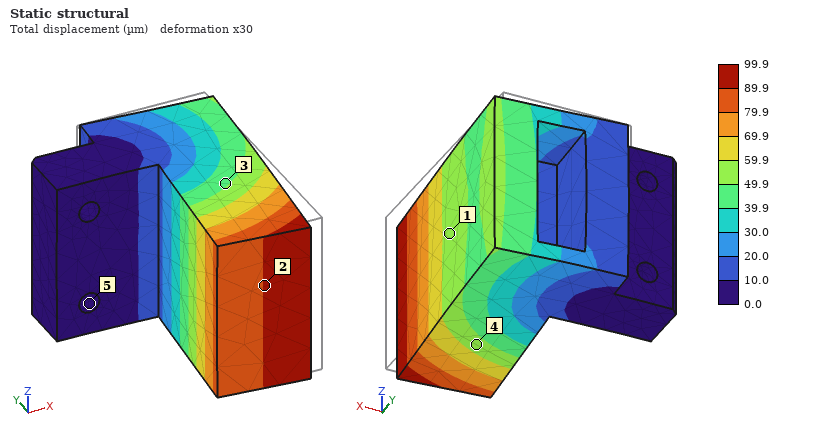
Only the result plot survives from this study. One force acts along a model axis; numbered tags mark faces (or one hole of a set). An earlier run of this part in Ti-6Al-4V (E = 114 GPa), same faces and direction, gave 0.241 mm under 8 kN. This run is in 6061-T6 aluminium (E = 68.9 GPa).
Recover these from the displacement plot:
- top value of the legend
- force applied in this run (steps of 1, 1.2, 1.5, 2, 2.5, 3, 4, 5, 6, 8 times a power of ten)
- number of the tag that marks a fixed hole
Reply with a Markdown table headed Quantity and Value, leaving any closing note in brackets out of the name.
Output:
| Quantity | Value |
|---|---|
| top value of the legend | 99.9 µm |
| force applied in this run | 2 kN |
| number of the tag that marks a fixed hole | 5 |
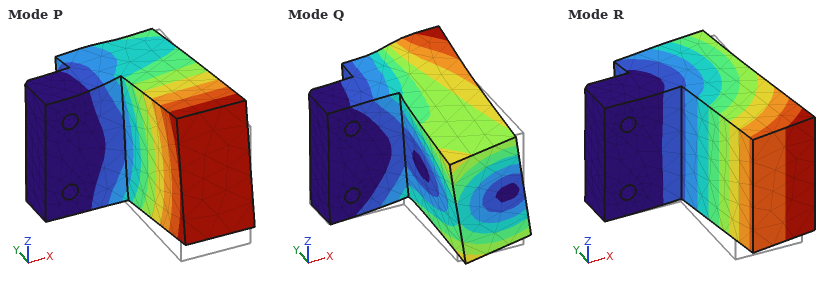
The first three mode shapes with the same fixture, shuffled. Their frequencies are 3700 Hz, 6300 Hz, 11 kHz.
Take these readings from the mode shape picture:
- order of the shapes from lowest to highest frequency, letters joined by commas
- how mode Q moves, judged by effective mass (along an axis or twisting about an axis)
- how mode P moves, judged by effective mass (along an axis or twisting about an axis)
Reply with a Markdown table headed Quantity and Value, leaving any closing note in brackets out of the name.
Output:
| Quantity | Value |
|---|---|
| order of the shapes from lowest to highest frequency, letters joined by commas | R, P, Q |
| how mode Q moves, judged by effective mass | along Z |
| how mode P moves, judged by effective mass | along Z |
